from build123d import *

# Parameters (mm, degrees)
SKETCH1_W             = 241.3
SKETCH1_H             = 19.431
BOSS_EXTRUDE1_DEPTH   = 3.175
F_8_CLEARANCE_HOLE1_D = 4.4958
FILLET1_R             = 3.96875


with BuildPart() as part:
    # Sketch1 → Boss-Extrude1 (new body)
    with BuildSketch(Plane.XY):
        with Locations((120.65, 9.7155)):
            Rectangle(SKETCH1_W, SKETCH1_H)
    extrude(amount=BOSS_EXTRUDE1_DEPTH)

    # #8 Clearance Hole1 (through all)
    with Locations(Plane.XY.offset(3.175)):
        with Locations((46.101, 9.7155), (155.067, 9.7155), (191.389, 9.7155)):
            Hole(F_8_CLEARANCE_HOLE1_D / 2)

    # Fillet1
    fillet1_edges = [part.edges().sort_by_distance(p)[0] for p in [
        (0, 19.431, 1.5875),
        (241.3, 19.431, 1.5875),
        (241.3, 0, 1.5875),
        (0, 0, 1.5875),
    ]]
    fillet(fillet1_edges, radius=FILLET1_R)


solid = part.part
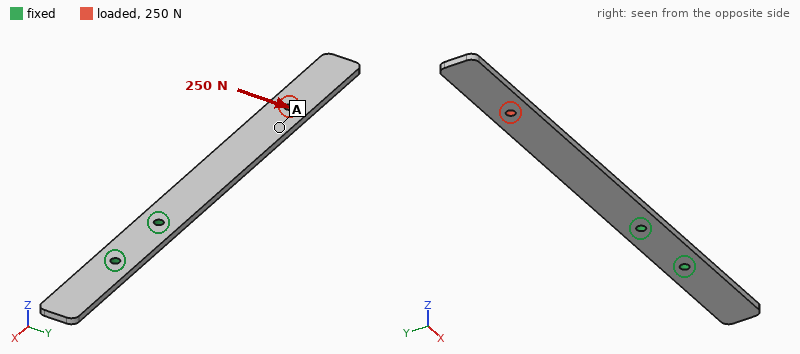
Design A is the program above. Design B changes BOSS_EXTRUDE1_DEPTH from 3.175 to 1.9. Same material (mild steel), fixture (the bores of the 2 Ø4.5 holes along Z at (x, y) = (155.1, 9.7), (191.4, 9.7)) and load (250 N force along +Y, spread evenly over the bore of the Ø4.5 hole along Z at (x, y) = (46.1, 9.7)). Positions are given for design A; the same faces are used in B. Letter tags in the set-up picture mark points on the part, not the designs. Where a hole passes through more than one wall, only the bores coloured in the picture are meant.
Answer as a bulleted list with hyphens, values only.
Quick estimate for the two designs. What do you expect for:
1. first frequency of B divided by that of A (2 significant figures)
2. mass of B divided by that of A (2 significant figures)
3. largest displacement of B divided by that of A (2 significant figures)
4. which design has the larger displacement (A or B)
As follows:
- 0.60
- 0.60
- 1.7
- B
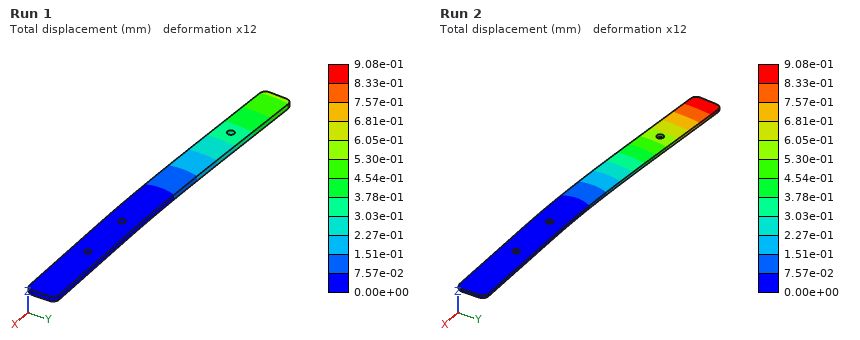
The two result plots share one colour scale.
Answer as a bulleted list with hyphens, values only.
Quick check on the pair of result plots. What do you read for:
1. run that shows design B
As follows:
- Run 2
